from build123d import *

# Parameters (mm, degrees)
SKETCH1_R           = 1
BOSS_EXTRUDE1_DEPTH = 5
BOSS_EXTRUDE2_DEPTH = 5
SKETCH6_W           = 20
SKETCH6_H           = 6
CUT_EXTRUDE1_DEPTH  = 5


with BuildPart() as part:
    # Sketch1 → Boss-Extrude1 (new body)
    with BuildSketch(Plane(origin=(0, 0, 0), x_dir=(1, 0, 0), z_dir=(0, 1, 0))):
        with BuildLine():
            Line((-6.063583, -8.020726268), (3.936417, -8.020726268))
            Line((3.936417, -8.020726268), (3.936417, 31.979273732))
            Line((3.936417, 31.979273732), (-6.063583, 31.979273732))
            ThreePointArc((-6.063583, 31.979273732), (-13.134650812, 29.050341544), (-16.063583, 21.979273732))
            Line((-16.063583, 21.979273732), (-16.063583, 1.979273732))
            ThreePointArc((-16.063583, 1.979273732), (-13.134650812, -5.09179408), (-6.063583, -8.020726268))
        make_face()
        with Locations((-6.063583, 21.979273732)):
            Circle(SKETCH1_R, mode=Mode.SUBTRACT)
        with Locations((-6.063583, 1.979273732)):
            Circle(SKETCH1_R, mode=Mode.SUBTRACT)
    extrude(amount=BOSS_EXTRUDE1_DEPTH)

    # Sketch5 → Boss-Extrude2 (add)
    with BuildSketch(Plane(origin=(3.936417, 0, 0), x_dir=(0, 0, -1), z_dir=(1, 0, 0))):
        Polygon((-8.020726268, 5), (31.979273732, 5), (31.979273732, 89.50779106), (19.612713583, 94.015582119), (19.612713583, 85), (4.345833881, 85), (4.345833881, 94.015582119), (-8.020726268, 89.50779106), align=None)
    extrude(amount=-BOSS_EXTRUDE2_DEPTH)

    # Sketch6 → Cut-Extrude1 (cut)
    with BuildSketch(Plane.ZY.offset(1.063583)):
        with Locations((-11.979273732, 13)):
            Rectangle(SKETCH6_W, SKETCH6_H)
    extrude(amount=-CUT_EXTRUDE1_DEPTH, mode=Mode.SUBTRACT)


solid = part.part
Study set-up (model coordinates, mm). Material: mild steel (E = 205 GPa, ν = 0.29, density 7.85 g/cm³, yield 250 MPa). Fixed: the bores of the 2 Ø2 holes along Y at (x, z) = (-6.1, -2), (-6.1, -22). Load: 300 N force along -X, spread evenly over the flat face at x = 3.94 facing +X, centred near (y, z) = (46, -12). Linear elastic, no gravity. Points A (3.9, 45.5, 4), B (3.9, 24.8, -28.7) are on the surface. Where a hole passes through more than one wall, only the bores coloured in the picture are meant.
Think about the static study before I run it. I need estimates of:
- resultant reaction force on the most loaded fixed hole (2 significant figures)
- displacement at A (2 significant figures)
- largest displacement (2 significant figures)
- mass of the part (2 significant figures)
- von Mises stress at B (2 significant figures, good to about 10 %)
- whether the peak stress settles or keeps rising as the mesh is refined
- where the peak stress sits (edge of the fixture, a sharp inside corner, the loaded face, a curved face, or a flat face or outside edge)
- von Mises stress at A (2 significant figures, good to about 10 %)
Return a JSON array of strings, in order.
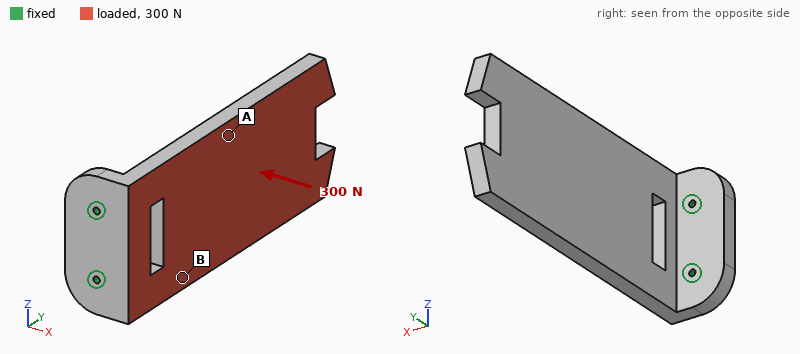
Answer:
["150 N", "0.22 mm", "0.58 mm", "160 g", "56 MPa", "keeps rising", "edge of the fixture", "21 MPa"]
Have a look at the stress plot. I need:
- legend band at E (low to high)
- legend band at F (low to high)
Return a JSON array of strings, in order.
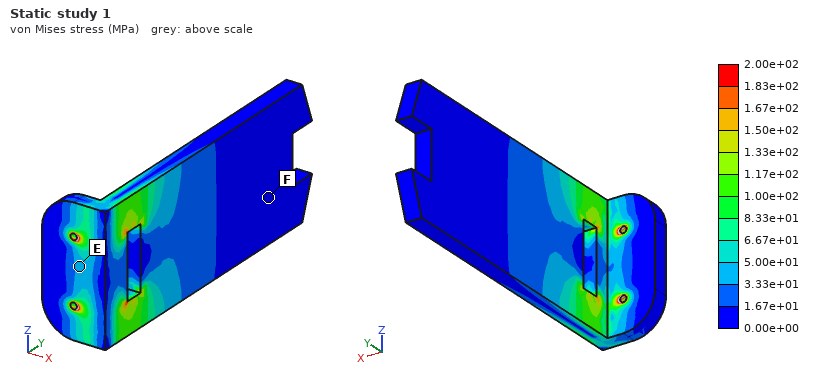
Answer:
["3.33e+01 to 5.00e+01 MPa", "0.00e+00 to 1.67e+01 MPa"]
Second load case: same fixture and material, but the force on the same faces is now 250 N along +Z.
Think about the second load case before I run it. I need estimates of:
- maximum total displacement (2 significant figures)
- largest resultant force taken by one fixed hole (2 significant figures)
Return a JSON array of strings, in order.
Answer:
["25 µm", "480 N"]
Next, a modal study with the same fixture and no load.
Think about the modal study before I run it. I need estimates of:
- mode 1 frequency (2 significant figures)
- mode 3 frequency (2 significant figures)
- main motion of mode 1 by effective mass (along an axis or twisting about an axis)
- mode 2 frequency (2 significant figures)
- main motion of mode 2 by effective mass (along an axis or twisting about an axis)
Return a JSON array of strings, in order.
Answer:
["390 Hz", "2300 Hz", "along X", "1600 Hz", "along Z"]
